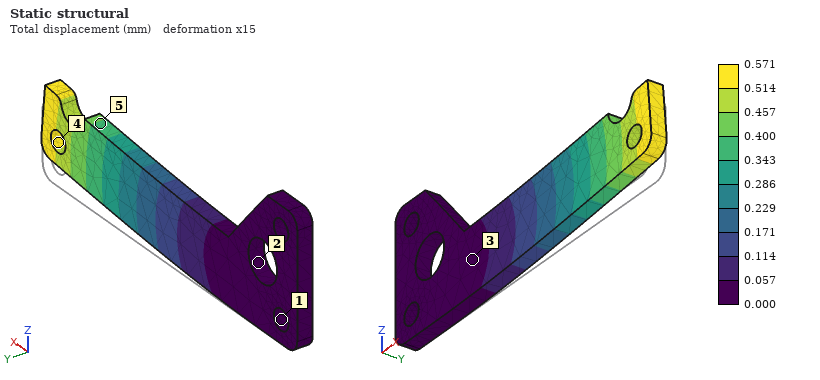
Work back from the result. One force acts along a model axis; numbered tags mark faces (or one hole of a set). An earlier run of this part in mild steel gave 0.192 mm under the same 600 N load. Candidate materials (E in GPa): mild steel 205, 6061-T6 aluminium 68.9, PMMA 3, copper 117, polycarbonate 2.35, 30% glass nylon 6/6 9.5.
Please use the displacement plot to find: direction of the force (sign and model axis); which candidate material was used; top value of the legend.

+Z
6061-T6 aluminium
0.571 mm
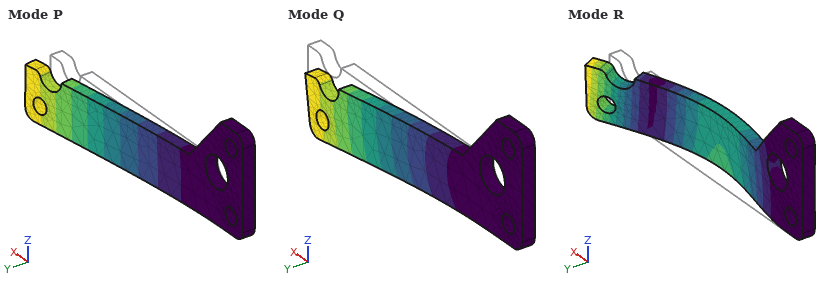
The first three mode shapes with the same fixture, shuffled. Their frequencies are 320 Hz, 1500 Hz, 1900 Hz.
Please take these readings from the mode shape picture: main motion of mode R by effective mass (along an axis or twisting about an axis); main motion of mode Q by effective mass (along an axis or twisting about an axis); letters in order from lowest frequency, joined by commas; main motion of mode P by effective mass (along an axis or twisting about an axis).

along Y
along Z
P, Q, R
along Y
